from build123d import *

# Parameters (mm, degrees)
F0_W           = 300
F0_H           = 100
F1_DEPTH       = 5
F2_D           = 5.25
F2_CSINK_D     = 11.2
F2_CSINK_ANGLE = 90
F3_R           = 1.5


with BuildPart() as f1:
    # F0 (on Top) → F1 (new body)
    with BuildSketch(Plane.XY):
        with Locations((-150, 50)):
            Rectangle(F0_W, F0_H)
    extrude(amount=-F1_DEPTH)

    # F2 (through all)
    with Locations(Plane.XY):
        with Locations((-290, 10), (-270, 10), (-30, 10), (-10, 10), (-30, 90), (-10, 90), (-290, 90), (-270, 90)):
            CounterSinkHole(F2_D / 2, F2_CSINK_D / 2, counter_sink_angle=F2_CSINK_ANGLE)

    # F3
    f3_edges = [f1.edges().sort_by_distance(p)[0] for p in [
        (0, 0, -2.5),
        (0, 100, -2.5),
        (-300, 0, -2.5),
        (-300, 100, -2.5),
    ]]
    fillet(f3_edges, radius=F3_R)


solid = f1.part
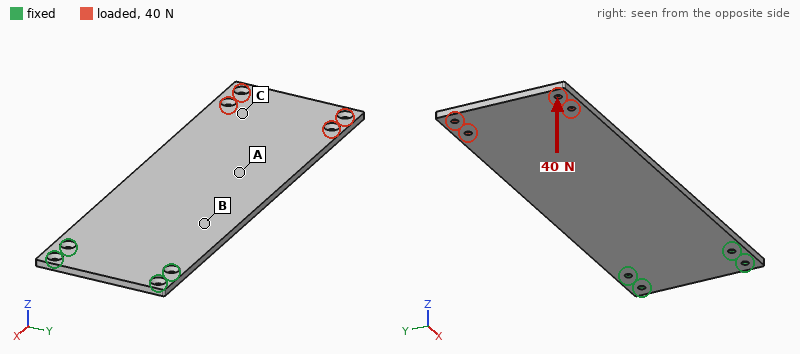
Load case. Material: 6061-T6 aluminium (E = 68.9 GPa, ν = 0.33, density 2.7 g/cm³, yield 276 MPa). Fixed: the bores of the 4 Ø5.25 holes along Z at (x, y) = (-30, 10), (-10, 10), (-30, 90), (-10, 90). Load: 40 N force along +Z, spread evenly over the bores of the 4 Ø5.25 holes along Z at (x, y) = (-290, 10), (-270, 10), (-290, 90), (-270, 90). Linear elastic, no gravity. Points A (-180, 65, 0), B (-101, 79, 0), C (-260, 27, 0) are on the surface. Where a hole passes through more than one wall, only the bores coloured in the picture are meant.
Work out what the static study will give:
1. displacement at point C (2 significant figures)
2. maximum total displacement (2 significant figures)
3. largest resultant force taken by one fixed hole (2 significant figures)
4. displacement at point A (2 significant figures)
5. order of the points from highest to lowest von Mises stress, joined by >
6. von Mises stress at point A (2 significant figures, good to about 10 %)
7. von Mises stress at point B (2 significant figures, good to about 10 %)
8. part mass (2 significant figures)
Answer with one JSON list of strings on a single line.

["2.8 mm", "3.6 mm", "360 N", "1.4 mm", "B > A > C", "9.6 MPa", "17 MPa", "400 g"]
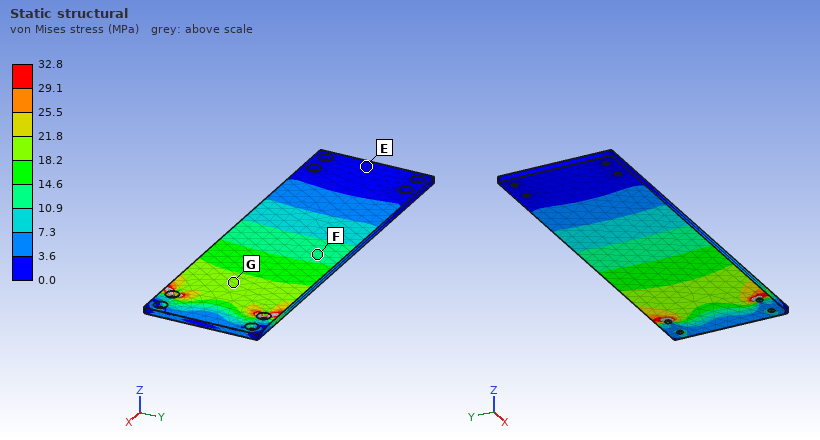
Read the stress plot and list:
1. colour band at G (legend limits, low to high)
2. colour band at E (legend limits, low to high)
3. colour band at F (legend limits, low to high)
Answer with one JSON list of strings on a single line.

["18.2 to 21.8 MPa", "0.0 to 3.6 MPa", "10.9 to 14.6 MPa"]
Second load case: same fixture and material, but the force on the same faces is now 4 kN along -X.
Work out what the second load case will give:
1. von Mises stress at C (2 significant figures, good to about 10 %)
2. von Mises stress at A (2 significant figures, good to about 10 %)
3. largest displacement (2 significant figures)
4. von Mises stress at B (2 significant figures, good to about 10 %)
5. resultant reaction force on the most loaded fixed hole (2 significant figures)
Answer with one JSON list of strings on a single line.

["8.1 MPa", "6.4 MPa", "3.1 mm", "6.2 MPa", "1.5 kN"]
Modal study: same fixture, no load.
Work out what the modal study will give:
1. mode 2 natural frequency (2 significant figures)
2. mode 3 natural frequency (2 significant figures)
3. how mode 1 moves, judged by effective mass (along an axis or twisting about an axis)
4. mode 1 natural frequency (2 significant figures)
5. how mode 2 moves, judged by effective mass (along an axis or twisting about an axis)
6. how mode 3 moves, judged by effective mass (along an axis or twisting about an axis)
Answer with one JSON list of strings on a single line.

["310 Hz", "330 Hz", "along Z", "53 Hz", "twisting about X", "along Z"]
